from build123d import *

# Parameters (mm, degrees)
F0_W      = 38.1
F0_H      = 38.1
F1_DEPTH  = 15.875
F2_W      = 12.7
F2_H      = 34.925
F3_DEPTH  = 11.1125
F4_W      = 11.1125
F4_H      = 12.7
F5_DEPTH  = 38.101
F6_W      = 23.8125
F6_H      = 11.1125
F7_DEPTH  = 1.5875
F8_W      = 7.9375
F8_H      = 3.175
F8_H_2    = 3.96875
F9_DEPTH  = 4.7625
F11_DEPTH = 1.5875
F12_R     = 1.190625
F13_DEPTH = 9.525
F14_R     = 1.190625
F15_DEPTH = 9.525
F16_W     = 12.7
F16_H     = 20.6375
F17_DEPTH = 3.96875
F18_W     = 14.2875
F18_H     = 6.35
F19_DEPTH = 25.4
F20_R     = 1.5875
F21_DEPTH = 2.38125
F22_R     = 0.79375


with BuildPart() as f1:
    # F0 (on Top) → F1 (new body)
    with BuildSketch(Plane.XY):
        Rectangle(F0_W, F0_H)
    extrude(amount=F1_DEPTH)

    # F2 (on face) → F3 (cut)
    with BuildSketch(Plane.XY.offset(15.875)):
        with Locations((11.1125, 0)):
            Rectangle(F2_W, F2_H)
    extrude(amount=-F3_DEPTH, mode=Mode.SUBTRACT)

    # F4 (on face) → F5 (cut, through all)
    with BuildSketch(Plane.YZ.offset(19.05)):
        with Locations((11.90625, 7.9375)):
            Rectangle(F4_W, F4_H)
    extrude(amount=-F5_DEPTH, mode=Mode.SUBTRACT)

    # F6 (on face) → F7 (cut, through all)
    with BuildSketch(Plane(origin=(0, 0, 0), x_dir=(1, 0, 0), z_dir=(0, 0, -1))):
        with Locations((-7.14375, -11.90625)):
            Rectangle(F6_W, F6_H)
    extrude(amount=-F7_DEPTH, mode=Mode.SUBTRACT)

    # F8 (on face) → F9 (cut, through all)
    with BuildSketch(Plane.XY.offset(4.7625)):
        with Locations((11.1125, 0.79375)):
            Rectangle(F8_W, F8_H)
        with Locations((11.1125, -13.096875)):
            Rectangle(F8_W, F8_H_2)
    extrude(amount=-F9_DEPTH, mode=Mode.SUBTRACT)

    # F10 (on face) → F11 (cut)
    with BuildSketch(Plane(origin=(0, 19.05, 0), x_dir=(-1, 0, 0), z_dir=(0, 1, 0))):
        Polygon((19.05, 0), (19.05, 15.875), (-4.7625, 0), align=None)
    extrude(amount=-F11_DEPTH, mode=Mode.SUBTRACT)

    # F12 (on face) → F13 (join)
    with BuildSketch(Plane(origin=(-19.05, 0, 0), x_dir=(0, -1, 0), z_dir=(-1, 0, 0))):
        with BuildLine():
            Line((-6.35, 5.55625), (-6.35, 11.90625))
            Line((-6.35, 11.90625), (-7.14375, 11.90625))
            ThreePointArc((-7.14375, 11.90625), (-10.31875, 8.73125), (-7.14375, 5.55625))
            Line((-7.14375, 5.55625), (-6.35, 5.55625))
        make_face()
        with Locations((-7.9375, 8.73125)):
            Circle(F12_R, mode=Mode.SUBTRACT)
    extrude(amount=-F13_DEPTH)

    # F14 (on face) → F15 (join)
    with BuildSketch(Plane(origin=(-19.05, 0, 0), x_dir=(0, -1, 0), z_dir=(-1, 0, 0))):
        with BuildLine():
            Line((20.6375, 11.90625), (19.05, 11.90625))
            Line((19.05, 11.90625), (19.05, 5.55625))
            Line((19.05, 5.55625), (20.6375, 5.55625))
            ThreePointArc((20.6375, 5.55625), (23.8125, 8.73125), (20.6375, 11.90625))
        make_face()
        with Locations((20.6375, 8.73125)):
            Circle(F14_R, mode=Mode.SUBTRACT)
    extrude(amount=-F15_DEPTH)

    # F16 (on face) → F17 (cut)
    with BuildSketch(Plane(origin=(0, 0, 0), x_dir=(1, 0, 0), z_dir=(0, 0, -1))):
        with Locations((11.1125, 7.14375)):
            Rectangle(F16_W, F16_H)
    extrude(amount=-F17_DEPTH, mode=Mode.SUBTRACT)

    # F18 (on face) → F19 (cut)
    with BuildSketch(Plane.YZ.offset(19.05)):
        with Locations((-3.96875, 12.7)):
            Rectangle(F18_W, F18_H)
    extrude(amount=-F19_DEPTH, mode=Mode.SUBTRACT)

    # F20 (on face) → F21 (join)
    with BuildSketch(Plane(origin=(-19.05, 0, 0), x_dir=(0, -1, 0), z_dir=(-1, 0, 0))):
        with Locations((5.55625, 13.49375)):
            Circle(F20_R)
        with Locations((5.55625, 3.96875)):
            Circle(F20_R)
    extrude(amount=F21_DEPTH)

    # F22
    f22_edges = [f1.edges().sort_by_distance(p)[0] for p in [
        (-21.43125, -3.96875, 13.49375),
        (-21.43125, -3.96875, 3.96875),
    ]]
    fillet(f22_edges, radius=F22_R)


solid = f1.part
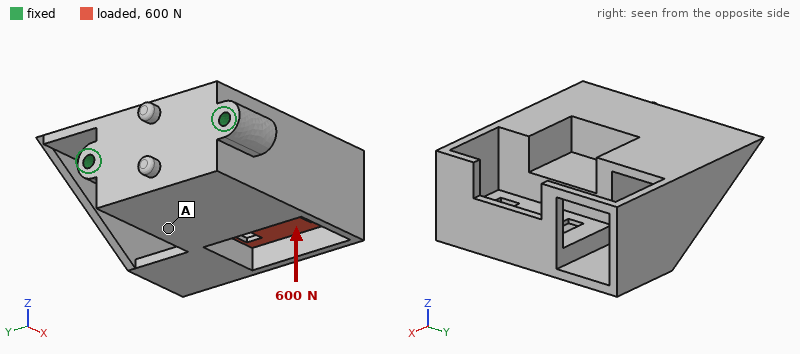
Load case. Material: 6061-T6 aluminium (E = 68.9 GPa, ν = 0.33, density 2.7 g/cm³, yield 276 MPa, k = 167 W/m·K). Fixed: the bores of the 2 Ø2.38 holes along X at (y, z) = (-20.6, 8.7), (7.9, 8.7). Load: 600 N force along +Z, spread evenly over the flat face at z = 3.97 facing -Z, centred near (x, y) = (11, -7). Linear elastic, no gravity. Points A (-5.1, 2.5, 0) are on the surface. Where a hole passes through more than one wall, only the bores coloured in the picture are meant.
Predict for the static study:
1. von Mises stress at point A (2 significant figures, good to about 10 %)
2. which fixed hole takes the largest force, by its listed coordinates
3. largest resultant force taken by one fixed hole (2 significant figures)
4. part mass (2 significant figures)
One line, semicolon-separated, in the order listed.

15 MPa; (-20.6, 8.7); 320 N; 31 g
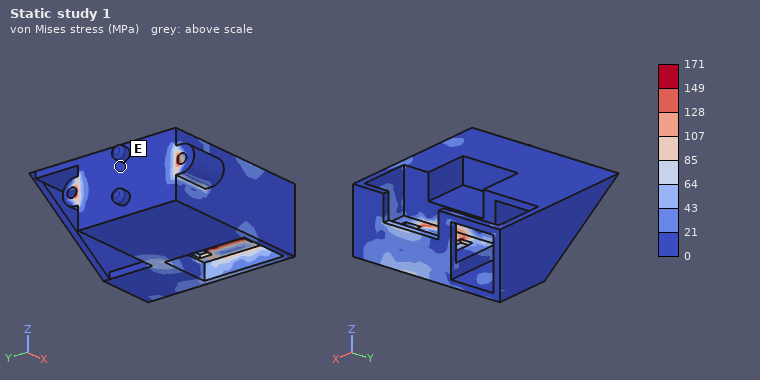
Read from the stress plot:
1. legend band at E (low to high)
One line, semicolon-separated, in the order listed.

0 to 21 MPa
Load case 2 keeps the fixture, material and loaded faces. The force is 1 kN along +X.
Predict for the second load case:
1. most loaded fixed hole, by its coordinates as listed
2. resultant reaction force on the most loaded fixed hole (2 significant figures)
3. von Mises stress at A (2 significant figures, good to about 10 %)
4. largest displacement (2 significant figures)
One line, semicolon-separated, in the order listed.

(-20.6, 8.7); 550 N; 6.4 MPa; 25 µm
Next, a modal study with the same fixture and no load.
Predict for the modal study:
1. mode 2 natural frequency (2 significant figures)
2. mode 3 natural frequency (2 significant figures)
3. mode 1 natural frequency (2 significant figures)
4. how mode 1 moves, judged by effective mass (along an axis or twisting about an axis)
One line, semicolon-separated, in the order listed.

6700 Hz; 8400 Hz; 4400 Hz; along Z
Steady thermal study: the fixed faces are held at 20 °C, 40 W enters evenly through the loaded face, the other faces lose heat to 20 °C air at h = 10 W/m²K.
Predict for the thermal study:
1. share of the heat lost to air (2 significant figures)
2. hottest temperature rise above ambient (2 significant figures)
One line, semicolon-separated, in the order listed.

3.4 %; 71 K
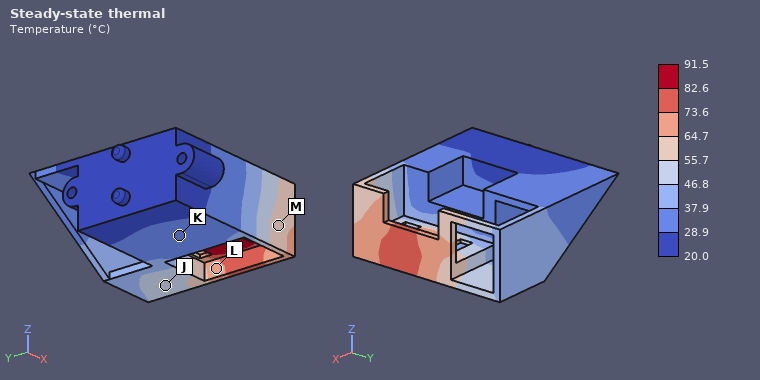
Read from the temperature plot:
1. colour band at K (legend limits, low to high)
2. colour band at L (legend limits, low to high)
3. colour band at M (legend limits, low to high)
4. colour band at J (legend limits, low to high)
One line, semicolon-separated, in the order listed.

28.9 to 37.9 °C; 64.7 to 73.6 °C; 55.7 to 64.7 °C; 46.8 to 55.7 °C
